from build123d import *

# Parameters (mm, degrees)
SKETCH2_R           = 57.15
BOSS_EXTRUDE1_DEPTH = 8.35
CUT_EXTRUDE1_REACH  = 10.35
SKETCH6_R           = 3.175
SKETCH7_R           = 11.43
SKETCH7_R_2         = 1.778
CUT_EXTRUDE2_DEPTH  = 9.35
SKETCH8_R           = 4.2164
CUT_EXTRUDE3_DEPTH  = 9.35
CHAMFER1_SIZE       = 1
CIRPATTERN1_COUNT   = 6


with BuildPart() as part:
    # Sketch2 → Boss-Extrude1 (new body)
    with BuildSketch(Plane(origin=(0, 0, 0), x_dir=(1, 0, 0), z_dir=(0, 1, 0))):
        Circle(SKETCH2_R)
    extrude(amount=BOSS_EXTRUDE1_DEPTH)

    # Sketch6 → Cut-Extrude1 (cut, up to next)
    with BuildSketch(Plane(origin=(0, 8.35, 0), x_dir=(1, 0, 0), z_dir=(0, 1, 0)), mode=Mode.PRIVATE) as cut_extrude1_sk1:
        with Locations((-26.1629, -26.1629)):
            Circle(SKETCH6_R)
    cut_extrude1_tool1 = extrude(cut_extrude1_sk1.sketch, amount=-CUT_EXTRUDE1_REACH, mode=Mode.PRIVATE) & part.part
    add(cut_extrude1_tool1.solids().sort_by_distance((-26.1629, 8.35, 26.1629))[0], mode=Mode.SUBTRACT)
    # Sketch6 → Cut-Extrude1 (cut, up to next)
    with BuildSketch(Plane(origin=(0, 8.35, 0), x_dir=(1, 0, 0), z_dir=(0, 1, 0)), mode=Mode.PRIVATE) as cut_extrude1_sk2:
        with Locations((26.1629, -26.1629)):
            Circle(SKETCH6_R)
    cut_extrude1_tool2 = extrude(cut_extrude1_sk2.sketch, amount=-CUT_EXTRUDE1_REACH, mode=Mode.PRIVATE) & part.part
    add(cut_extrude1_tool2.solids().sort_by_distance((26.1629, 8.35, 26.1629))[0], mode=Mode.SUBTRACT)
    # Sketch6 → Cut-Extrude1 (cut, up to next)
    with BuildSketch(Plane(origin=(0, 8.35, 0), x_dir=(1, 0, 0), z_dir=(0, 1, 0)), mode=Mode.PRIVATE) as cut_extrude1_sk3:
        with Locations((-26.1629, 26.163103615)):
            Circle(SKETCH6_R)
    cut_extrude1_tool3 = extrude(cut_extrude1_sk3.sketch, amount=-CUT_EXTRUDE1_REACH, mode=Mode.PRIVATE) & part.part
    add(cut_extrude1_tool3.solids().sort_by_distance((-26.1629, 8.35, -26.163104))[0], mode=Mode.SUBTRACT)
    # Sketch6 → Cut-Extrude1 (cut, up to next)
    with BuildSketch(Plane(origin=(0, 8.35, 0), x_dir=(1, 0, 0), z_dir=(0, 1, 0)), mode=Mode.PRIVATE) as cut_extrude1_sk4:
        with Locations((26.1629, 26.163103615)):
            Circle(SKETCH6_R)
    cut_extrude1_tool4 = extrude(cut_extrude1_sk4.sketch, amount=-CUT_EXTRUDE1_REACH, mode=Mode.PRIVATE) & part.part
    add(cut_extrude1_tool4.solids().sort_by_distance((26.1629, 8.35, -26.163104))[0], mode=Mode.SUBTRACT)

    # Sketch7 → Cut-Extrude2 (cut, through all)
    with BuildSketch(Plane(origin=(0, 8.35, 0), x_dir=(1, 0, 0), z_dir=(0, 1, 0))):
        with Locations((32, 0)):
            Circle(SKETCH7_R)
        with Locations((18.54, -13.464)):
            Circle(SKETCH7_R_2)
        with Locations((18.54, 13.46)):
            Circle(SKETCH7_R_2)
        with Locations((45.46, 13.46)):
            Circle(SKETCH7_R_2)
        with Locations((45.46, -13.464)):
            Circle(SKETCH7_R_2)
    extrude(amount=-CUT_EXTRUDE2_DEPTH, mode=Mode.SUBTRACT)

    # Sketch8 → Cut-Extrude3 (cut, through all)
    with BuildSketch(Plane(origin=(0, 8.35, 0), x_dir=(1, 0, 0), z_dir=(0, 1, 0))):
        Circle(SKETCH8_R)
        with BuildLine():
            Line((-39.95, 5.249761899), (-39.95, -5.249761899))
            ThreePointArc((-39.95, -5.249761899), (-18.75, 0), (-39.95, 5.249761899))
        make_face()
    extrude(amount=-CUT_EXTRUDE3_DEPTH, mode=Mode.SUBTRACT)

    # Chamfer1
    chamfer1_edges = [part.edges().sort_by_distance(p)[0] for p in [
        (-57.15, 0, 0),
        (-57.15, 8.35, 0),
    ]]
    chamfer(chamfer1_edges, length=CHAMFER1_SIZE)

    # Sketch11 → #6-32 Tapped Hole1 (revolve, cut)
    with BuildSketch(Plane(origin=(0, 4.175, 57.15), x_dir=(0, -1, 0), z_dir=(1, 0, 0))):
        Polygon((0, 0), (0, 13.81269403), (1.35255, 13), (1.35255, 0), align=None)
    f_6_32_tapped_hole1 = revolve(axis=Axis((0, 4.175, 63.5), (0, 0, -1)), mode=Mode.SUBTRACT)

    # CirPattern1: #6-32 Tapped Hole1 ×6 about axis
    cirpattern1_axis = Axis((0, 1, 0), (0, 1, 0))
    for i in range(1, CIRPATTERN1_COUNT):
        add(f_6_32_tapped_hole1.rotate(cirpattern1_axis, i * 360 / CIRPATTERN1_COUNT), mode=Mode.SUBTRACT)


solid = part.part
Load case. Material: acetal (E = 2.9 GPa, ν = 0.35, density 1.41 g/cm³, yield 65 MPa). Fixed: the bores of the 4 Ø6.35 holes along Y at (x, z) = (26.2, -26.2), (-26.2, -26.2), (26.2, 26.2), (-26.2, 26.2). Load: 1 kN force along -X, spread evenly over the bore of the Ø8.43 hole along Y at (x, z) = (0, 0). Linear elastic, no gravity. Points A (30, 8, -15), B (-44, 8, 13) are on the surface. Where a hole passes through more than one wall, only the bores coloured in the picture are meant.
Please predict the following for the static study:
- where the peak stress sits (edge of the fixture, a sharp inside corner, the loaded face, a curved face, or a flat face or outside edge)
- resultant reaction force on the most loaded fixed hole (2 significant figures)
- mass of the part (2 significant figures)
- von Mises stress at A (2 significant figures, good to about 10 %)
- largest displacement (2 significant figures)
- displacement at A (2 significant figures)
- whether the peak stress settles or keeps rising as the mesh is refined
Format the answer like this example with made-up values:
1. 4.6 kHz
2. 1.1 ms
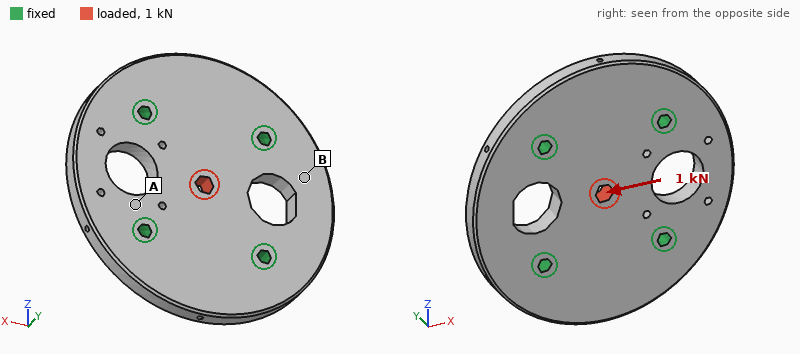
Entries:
1. a sharp inside corner
2. 290 N
3. 110 g
4. 1.1 MPa
5. 35 µm
6. 7.3 µm
7. keeps rising
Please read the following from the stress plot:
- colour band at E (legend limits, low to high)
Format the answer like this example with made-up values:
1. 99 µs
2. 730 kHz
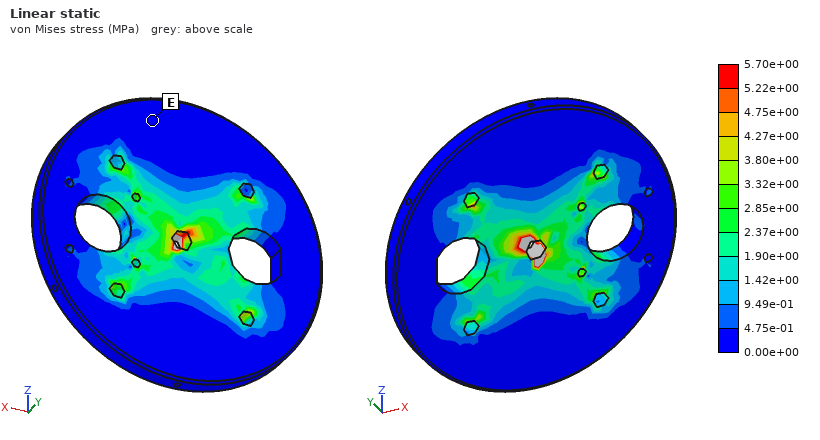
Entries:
1. 0.00e+00 to 4.75e-01 MPa
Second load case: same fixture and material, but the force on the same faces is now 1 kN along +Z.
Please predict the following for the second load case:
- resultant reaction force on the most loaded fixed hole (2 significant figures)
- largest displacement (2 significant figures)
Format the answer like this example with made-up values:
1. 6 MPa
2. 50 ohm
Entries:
1. 260 N
2. 30 µm
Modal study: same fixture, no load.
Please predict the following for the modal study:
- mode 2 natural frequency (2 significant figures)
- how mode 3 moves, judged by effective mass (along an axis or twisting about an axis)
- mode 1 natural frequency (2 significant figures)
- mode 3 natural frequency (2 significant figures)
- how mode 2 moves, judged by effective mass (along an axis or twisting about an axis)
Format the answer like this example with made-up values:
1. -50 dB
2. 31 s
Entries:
1. 1900 Hz
2. twisting about X
3. 1800 Hz
4. 2000 Hz
5. twisting about Z
